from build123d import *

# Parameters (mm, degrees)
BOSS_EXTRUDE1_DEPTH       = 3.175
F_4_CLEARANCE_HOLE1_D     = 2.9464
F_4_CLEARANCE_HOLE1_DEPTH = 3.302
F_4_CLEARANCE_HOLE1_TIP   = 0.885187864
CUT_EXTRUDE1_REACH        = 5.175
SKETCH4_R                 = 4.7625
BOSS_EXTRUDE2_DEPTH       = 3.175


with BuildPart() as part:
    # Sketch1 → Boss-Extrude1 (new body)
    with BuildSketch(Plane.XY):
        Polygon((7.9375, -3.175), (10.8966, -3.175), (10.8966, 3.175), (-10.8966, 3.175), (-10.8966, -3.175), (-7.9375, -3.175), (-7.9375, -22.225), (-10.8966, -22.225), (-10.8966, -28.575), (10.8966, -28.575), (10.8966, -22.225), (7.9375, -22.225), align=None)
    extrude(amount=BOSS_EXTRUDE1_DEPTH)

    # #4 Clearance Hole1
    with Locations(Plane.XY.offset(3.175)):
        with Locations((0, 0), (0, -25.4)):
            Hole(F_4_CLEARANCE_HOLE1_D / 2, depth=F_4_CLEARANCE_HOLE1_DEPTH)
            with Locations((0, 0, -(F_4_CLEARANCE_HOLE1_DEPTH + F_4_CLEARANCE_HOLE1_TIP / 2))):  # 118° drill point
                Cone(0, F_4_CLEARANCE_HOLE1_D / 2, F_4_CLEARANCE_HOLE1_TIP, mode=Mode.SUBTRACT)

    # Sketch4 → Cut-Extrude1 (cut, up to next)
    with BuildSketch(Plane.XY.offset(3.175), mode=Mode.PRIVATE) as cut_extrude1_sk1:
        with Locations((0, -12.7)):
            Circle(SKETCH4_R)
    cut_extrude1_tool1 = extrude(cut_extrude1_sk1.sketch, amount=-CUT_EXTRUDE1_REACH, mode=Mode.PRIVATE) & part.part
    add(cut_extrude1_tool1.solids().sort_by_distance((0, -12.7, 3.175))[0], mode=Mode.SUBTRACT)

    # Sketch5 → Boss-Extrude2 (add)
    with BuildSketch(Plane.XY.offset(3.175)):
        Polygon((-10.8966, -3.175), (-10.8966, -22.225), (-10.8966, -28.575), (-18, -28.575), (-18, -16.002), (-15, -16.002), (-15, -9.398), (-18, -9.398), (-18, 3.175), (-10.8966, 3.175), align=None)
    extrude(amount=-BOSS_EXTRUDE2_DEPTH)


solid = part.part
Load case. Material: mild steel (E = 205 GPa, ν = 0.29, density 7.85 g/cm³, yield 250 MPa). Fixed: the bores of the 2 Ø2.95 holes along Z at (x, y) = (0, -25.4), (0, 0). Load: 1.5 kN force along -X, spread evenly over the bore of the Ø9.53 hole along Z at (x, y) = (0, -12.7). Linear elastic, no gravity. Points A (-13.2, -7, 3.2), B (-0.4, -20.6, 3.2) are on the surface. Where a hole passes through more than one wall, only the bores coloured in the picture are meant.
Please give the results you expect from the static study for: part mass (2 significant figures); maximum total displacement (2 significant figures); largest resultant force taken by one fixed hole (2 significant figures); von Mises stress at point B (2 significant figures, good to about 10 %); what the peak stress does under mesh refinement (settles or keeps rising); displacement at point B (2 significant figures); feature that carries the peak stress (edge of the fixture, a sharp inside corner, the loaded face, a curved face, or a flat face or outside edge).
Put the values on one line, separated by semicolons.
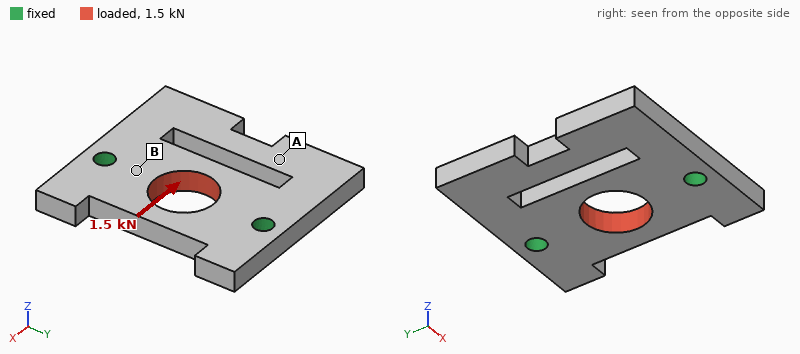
17 g; 3.9 µm; 750 N; 38 MPa; keeps rising; 1.5 µm; edge of the fixture
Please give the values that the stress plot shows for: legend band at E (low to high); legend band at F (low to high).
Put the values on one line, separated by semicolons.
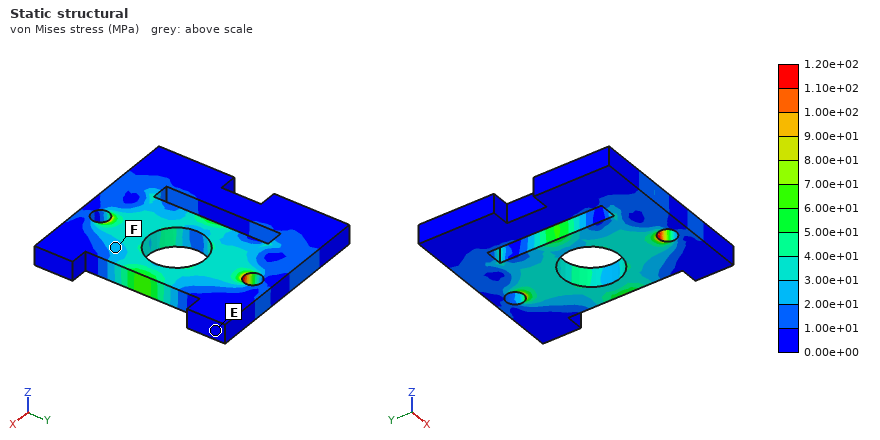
0.00e+00 to 1.00e+01 MPa; 2.00e+01 to 3.00e+01 MPa
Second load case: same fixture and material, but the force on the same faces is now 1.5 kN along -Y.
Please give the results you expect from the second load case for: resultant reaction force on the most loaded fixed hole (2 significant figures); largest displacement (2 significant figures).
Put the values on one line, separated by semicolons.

750 N; 1.5 µm
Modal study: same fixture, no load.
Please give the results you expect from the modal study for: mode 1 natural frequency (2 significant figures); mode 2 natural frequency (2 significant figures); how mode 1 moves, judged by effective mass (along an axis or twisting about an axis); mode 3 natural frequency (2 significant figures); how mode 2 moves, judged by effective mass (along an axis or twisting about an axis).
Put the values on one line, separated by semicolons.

6500 Hz; 11 kHz; along Z; 20 kHz; twisting about X
